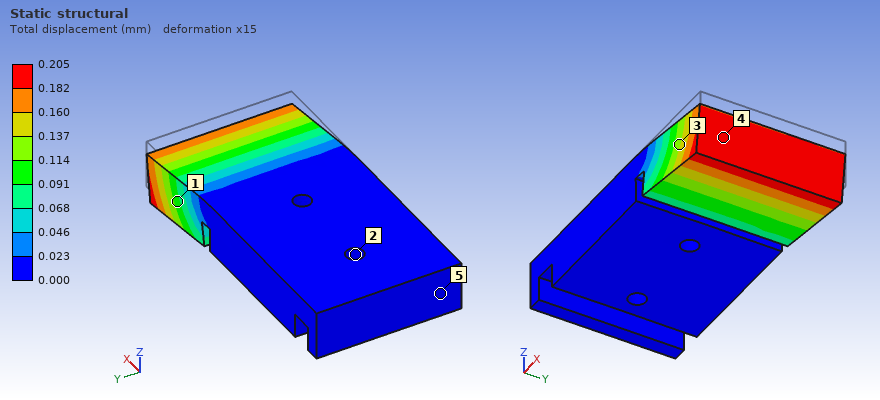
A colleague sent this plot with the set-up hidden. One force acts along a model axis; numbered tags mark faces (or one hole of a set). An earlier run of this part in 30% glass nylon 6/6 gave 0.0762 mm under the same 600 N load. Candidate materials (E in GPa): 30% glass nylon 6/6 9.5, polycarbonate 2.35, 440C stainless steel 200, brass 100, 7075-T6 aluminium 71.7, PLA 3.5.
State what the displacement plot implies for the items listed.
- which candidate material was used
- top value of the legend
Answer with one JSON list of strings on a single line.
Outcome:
["PLA", "0.205 mm"]
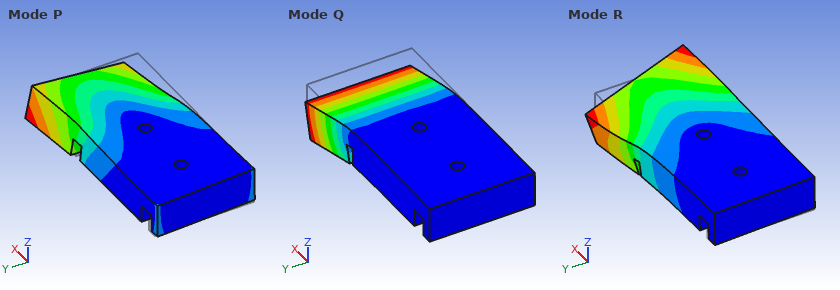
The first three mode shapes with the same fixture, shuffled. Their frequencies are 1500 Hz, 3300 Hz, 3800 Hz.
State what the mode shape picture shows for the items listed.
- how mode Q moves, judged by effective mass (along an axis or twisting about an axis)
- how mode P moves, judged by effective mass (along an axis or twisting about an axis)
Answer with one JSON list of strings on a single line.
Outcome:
["along Z", "along Y"]
